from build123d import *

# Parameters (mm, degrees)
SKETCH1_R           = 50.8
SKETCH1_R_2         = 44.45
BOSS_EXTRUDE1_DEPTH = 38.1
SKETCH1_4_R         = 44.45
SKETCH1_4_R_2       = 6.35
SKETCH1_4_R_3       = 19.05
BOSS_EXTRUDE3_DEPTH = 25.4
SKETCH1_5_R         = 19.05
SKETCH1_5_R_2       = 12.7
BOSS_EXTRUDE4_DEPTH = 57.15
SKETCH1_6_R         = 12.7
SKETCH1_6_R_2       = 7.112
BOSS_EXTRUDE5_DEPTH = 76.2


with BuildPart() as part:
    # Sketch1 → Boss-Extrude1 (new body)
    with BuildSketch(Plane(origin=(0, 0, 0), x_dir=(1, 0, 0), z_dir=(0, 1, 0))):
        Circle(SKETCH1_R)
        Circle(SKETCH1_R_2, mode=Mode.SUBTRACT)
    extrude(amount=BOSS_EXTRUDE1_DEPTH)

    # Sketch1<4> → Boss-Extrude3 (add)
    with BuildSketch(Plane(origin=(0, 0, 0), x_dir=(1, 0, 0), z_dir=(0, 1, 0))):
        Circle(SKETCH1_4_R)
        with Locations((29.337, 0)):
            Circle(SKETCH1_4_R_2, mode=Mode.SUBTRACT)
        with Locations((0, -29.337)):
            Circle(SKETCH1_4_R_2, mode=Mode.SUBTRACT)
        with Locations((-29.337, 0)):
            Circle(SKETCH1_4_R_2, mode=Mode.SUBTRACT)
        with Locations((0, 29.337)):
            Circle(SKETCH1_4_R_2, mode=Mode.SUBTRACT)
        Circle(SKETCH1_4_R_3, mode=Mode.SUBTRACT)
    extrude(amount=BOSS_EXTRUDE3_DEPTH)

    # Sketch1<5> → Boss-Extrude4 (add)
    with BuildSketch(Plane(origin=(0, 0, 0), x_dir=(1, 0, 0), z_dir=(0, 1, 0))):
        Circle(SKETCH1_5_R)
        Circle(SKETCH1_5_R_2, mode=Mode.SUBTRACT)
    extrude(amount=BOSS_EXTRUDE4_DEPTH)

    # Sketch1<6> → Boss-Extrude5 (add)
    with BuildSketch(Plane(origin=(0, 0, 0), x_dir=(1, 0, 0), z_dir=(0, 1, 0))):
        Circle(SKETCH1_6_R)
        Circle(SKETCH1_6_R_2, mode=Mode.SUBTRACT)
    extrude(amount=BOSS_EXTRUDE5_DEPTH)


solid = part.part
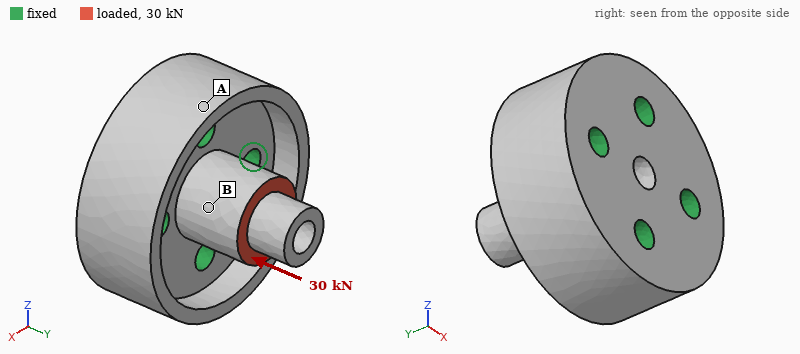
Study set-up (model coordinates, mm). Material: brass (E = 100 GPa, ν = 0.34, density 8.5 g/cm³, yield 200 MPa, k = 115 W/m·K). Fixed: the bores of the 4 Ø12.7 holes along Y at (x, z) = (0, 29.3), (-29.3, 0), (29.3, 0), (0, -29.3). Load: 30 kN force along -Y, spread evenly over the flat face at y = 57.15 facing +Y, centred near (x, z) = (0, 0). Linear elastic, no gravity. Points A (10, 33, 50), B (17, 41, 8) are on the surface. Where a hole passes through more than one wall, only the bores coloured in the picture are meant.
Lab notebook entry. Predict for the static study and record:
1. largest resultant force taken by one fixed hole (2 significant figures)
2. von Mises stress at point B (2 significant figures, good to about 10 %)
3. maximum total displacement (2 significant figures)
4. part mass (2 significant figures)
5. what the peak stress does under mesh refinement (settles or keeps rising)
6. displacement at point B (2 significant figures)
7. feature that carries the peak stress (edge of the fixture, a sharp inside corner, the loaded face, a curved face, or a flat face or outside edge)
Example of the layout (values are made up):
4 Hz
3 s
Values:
8.1 kN
31 MPa
16 µm
2.1 kg
keeps rising
9.5 µm
edge of the fixture
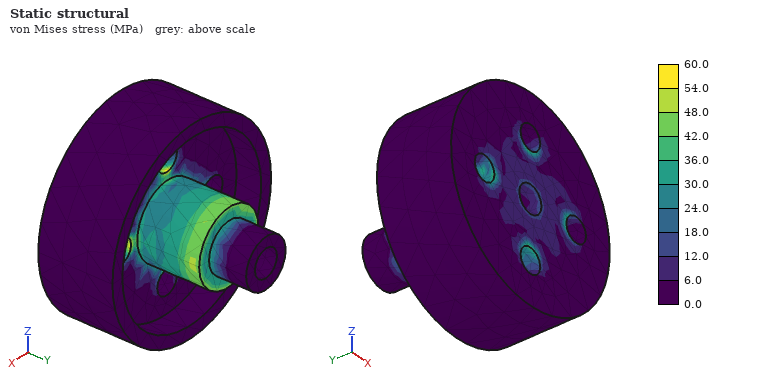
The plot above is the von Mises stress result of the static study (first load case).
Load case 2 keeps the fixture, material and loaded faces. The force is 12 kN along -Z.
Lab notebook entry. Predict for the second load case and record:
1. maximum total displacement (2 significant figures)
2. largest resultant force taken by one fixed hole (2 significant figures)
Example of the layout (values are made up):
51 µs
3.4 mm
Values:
54 µm
9.8 kN
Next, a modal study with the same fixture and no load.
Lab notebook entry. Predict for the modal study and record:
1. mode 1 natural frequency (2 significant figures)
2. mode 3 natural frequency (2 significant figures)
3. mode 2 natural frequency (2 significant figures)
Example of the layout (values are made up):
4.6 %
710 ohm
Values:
6300 Hz
10 kHz
6400 Hz
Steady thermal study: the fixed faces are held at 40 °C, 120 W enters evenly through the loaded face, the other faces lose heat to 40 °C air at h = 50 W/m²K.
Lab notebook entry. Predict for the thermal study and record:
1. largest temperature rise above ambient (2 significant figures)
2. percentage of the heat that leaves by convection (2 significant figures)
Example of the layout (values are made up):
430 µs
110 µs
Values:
42 K
10 %
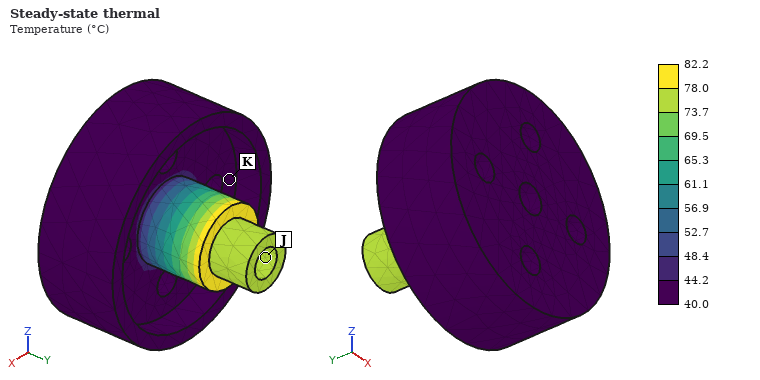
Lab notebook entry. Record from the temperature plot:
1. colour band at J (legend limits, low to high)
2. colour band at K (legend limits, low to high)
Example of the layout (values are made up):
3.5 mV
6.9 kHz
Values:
73.7 to 78.0 °C
40.0 to 44.2 °C
